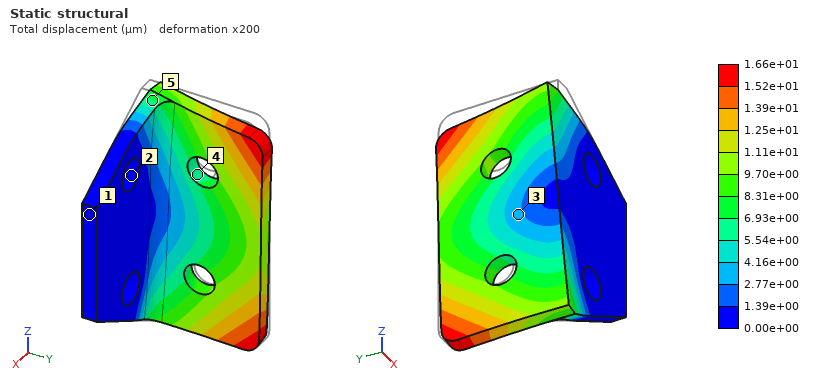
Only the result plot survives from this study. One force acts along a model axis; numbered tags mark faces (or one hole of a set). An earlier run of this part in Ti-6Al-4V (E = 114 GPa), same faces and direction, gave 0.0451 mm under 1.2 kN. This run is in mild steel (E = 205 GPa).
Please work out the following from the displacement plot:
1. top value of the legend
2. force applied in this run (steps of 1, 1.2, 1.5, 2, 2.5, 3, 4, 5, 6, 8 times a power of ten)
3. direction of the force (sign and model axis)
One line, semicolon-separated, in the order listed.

1.66e+01 µm; 800 N; -Z
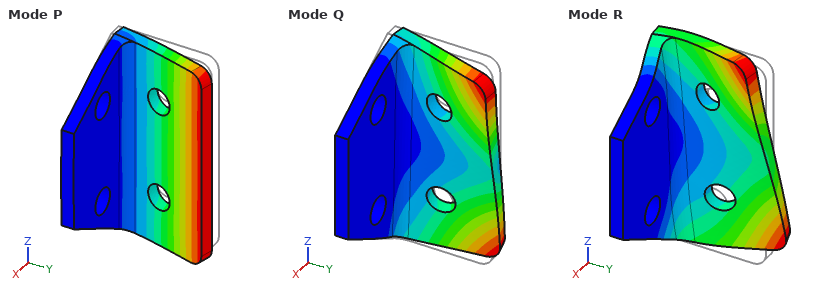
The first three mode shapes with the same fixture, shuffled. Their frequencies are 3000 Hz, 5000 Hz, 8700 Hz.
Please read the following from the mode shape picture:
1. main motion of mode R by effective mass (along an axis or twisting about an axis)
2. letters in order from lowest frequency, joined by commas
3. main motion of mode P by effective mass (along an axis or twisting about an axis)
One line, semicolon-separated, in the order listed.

along Z; P, Q, R; along X
